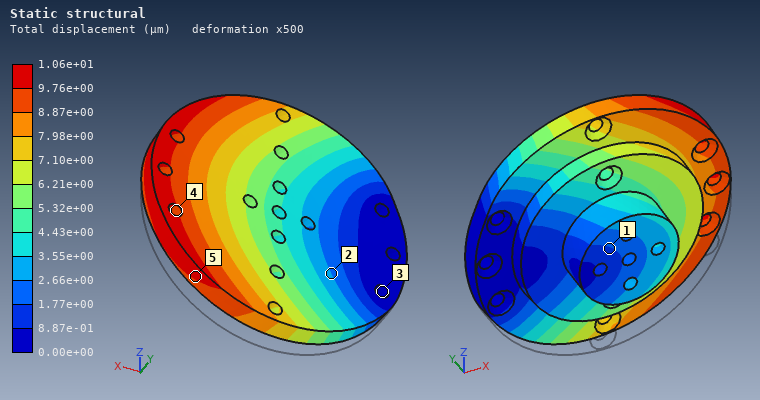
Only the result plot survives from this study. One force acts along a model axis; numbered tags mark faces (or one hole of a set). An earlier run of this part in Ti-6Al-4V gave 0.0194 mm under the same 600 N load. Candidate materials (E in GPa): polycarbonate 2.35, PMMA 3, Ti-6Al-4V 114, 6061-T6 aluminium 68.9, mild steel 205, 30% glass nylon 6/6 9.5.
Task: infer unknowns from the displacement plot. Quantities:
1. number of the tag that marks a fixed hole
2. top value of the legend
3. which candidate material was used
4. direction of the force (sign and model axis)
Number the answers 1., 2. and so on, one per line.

1. 3
2. 1.06e+01 µm
3. mild steel
4. +Z
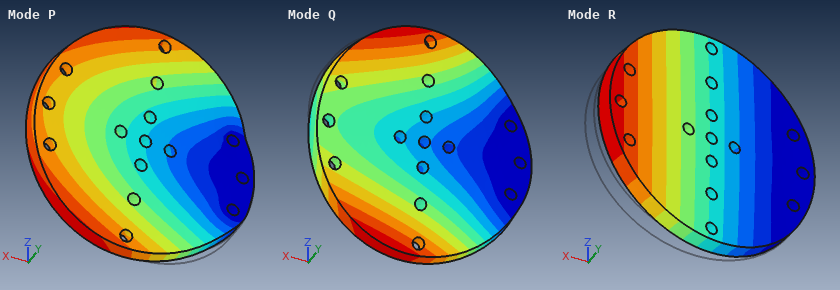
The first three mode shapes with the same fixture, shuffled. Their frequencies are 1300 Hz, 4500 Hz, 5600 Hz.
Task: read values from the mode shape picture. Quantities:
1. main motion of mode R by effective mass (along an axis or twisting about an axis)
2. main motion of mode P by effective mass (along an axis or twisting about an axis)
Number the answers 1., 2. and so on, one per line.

1. along Y
2. along Z
